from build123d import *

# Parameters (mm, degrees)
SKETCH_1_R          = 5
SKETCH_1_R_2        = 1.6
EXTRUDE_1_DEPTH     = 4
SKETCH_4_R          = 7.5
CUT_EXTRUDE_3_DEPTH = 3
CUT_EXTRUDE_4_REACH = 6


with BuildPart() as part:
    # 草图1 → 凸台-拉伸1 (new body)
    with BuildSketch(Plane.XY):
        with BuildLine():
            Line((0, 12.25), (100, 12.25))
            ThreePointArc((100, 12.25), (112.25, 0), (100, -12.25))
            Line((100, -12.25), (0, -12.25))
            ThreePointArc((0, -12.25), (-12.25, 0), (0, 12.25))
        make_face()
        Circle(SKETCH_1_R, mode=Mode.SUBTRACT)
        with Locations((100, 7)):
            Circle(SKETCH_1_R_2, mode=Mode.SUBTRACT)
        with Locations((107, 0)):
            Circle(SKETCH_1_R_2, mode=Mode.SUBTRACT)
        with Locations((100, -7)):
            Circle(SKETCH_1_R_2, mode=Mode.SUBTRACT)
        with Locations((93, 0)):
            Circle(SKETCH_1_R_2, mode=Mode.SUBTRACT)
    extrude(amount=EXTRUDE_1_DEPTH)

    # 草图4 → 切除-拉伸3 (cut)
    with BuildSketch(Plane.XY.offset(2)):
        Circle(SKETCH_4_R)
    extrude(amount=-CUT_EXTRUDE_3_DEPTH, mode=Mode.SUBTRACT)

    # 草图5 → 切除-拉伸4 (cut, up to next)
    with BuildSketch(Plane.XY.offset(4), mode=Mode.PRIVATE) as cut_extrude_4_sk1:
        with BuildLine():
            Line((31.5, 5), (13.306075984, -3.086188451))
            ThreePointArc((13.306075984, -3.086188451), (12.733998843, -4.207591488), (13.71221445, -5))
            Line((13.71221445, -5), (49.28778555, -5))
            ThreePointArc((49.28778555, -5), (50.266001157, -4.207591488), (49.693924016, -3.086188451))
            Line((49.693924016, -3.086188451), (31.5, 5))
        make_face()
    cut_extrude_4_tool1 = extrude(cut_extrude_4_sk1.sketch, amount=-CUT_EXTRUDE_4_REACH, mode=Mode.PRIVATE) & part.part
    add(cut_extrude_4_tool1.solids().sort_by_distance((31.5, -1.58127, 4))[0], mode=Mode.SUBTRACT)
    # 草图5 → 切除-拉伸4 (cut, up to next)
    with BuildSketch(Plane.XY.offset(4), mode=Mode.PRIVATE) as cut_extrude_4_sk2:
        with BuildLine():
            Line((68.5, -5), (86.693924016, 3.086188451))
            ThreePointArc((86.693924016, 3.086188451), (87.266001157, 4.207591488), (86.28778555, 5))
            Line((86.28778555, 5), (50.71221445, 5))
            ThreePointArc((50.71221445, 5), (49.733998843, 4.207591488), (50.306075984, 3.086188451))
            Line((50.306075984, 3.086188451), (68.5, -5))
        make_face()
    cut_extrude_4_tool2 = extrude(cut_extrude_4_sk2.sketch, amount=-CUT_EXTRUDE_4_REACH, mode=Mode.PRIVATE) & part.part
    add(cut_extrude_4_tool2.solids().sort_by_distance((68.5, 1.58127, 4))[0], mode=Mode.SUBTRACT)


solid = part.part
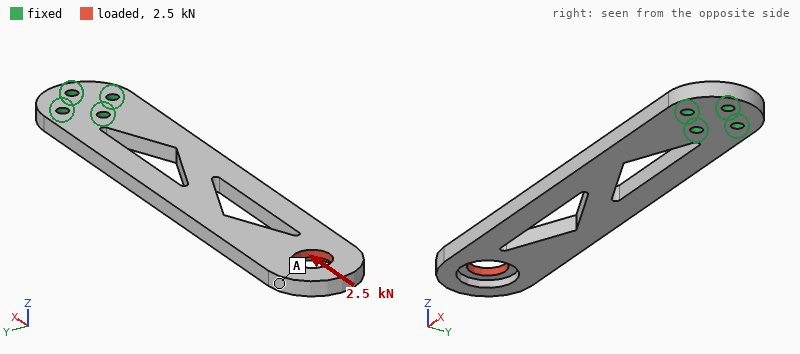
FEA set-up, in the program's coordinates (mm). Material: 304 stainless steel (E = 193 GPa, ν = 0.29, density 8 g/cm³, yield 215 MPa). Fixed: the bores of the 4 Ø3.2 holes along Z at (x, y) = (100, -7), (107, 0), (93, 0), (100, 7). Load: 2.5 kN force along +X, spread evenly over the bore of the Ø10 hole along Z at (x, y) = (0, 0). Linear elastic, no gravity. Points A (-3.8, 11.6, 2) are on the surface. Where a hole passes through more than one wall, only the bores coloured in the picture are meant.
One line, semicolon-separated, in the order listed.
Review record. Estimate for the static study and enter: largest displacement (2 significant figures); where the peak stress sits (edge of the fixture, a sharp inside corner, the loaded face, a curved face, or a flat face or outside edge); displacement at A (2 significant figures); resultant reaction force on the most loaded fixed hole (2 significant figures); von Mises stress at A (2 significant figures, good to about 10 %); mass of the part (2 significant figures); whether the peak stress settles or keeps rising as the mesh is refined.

0.73 mm; a sharp inside corner; 0.63 mm; 870 N; 15 MPa; 74 g; keeps rising
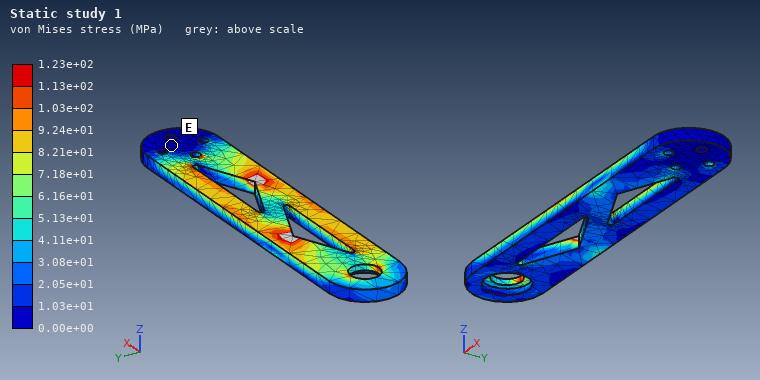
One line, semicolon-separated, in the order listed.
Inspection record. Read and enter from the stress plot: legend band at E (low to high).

0.00e+00 to 1.03e+01 MPa
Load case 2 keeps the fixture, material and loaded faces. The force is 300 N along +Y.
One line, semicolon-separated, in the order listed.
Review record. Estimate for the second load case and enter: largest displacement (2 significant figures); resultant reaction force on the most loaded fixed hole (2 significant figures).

0.16 mm; 1.4 kN
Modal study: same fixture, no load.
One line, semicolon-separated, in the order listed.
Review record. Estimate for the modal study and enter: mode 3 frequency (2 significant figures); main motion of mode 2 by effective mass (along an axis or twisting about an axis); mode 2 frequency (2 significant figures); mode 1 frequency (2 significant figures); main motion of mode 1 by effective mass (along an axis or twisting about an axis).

1800 Hz; along Y; 1600 Hz; 300 Hz; along Z
